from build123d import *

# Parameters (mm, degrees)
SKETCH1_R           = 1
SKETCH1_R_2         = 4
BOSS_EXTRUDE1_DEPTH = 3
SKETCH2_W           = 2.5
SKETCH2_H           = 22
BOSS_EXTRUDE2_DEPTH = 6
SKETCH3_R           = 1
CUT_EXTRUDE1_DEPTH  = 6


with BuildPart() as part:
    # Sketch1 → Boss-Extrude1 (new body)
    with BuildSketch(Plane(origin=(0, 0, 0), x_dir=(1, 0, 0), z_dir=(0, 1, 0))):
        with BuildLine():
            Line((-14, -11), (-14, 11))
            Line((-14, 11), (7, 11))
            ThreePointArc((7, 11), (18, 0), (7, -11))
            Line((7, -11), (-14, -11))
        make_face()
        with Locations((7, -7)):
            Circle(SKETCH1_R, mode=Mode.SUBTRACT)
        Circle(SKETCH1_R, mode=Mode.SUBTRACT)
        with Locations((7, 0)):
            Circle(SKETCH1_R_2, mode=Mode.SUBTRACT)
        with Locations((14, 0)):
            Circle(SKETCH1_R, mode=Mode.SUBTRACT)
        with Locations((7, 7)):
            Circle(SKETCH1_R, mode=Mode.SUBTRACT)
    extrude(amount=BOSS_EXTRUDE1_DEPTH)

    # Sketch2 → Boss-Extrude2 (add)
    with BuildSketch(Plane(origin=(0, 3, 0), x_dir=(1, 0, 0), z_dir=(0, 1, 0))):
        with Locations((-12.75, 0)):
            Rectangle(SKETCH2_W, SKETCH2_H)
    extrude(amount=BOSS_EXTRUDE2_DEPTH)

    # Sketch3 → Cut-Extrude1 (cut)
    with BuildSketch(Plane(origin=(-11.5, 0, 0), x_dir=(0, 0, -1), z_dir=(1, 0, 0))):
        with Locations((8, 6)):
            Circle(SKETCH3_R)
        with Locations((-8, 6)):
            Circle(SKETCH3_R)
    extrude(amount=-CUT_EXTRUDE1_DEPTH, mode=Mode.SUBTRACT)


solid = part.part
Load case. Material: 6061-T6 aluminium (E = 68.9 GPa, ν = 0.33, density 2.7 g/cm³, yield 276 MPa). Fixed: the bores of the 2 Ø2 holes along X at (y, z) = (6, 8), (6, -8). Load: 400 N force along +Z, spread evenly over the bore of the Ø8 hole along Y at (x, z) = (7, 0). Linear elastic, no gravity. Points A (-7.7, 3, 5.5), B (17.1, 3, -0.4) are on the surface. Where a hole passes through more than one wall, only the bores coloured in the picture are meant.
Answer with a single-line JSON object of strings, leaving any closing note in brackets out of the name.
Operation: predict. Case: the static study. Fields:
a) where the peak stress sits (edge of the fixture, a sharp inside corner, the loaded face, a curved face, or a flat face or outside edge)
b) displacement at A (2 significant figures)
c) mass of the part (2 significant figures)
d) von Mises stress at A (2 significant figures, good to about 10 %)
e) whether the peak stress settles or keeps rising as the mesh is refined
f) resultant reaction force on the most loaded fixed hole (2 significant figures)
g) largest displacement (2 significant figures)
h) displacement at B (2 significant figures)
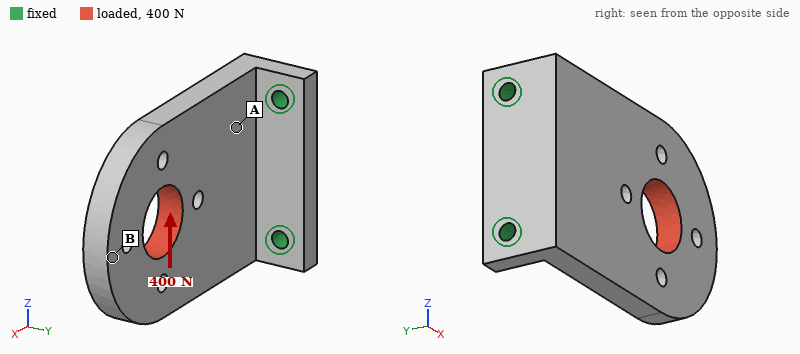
{"where the peak stress sits": "edge of the fixture", "displacement at A": "16 µm", "mass of the part": "5.6 g", "von Mises stress at A": "42 MPa", "whether the peak stress settles or keeps rising as the mesh is refined": "keeps rising", "resultant reaction force on the most loaded fixed hole": "520 N", "largest displacement": "70 µm", "displacement at B": "68 µm"}
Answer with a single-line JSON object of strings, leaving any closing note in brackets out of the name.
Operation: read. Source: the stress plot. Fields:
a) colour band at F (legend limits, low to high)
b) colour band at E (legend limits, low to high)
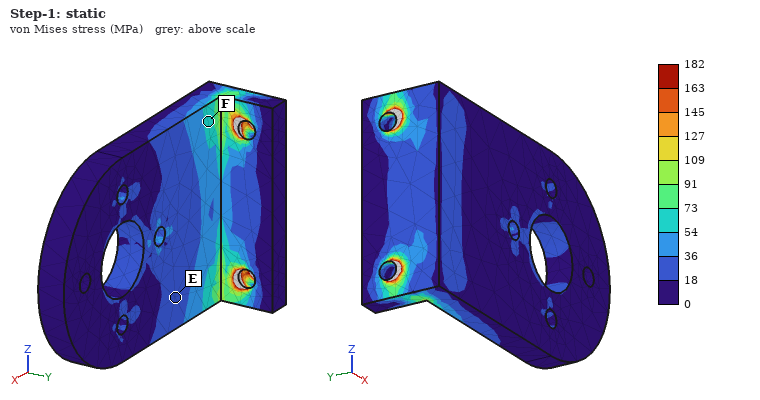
{"colour band at F": "54 to 73 MPa", "colour band at E": "18 to 36 MPa"}
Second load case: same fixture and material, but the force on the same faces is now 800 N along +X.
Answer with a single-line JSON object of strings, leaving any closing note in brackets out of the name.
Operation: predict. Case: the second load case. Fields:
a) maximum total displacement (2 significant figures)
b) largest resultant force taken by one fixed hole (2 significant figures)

{"maximum total displacement": "0.16 mm", "largest resultant force taken by one fixed hole": "400 N"}
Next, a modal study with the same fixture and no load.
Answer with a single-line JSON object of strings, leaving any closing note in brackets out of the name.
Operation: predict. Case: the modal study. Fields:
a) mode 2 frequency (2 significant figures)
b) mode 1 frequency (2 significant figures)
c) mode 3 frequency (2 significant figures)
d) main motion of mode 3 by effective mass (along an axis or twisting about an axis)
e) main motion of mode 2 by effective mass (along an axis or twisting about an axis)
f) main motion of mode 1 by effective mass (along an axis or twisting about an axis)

{"mode 2 frequency": "7300 Hz", "mode 1 frequency": "2200 Hz", "mode 3 frequency": "9700 Hz", "main motion of mode 3 by effective mass": "along Z", "main motion of mode 2 by effective mass": "along Z", "main motion of mode 1 by effective mass": "along Y"}
